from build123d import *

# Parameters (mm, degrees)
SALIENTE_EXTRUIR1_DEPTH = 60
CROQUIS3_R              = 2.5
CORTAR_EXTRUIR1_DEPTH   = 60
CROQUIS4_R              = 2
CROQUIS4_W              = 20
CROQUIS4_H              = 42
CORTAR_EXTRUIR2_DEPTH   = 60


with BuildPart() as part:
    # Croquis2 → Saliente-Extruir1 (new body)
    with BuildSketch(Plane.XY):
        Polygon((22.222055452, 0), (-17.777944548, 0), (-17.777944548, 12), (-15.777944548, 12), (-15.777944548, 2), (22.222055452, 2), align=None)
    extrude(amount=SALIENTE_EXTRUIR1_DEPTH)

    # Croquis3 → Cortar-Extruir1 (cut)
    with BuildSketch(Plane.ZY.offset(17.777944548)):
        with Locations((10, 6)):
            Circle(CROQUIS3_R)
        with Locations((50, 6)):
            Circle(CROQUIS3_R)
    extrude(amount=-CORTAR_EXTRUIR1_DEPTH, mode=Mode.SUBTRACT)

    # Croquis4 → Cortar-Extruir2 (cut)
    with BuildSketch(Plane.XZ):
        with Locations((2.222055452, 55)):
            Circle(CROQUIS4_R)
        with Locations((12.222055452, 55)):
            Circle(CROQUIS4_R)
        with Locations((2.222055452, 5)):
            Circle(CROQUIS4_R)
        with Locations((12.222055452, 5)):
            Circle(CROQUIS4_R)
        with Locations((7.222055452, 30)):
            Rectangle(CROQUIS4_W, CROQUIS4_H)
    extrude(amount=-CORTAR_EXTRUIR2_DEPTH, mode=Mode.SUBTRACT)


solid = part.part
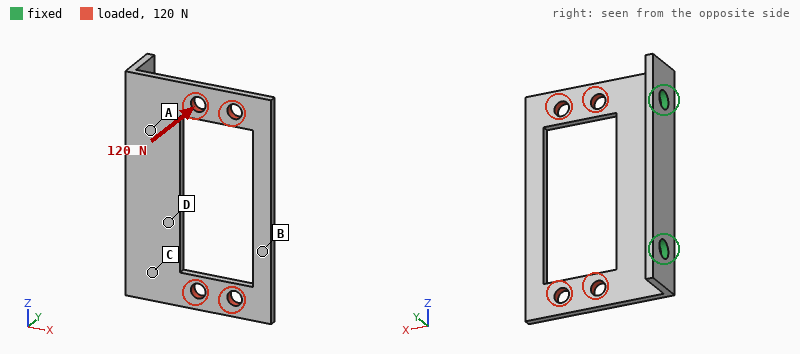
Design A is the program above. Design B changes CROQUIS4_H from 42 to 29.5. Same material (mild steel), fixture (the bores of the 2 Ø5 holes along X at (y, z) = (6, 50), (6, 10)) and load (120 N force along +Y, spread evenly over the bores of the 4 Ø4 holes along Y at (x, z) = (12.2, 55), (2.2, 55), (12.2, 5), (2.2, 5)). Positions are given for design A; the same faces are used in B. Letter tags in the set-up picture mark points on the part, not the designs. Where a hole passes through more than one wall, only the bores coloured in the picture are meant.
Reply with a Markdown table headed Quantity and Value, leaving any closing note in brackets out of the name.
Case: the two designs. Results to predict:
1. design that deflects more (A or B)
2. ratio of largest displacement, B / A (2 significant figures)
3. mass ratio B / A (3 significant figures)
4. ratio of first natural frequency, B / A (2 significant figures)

| Quantity | Value |
|---|---|
| design that deflects more | A |
| ratio of largest displacement, B / A | 0.77 |
| mass ratio B / A | 1.12 |
| ratio of first natural frequency, B / A | 1.1 |
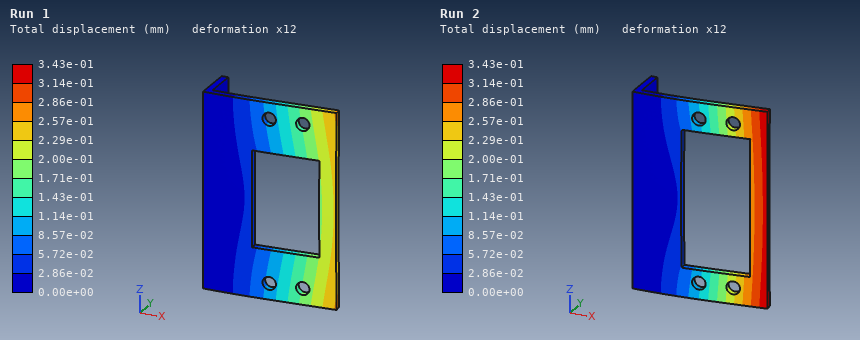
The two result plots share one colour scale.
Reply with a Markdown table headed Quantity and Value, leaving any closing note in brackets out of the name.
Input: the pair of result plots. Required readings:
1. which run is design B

| Quantity | Value |
|---|---|
| which run is design B | Run 1 |
